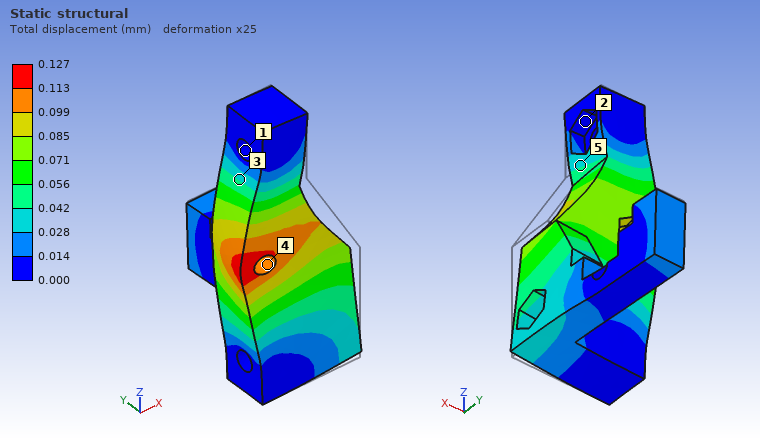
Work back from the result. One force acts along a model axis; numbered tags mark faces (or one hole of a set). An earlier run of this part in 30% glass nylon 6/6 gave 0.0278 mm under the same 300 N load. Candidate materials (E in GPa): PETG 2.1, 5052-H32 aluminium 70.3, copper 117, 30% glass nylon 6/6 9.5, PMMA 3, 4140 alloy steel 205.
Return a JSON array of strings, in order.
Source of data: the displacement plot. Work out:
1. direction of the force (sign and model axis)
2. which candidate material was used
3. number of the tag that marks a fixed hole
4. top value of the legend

["-X", "PETG", "1", "0.127 mm"]
